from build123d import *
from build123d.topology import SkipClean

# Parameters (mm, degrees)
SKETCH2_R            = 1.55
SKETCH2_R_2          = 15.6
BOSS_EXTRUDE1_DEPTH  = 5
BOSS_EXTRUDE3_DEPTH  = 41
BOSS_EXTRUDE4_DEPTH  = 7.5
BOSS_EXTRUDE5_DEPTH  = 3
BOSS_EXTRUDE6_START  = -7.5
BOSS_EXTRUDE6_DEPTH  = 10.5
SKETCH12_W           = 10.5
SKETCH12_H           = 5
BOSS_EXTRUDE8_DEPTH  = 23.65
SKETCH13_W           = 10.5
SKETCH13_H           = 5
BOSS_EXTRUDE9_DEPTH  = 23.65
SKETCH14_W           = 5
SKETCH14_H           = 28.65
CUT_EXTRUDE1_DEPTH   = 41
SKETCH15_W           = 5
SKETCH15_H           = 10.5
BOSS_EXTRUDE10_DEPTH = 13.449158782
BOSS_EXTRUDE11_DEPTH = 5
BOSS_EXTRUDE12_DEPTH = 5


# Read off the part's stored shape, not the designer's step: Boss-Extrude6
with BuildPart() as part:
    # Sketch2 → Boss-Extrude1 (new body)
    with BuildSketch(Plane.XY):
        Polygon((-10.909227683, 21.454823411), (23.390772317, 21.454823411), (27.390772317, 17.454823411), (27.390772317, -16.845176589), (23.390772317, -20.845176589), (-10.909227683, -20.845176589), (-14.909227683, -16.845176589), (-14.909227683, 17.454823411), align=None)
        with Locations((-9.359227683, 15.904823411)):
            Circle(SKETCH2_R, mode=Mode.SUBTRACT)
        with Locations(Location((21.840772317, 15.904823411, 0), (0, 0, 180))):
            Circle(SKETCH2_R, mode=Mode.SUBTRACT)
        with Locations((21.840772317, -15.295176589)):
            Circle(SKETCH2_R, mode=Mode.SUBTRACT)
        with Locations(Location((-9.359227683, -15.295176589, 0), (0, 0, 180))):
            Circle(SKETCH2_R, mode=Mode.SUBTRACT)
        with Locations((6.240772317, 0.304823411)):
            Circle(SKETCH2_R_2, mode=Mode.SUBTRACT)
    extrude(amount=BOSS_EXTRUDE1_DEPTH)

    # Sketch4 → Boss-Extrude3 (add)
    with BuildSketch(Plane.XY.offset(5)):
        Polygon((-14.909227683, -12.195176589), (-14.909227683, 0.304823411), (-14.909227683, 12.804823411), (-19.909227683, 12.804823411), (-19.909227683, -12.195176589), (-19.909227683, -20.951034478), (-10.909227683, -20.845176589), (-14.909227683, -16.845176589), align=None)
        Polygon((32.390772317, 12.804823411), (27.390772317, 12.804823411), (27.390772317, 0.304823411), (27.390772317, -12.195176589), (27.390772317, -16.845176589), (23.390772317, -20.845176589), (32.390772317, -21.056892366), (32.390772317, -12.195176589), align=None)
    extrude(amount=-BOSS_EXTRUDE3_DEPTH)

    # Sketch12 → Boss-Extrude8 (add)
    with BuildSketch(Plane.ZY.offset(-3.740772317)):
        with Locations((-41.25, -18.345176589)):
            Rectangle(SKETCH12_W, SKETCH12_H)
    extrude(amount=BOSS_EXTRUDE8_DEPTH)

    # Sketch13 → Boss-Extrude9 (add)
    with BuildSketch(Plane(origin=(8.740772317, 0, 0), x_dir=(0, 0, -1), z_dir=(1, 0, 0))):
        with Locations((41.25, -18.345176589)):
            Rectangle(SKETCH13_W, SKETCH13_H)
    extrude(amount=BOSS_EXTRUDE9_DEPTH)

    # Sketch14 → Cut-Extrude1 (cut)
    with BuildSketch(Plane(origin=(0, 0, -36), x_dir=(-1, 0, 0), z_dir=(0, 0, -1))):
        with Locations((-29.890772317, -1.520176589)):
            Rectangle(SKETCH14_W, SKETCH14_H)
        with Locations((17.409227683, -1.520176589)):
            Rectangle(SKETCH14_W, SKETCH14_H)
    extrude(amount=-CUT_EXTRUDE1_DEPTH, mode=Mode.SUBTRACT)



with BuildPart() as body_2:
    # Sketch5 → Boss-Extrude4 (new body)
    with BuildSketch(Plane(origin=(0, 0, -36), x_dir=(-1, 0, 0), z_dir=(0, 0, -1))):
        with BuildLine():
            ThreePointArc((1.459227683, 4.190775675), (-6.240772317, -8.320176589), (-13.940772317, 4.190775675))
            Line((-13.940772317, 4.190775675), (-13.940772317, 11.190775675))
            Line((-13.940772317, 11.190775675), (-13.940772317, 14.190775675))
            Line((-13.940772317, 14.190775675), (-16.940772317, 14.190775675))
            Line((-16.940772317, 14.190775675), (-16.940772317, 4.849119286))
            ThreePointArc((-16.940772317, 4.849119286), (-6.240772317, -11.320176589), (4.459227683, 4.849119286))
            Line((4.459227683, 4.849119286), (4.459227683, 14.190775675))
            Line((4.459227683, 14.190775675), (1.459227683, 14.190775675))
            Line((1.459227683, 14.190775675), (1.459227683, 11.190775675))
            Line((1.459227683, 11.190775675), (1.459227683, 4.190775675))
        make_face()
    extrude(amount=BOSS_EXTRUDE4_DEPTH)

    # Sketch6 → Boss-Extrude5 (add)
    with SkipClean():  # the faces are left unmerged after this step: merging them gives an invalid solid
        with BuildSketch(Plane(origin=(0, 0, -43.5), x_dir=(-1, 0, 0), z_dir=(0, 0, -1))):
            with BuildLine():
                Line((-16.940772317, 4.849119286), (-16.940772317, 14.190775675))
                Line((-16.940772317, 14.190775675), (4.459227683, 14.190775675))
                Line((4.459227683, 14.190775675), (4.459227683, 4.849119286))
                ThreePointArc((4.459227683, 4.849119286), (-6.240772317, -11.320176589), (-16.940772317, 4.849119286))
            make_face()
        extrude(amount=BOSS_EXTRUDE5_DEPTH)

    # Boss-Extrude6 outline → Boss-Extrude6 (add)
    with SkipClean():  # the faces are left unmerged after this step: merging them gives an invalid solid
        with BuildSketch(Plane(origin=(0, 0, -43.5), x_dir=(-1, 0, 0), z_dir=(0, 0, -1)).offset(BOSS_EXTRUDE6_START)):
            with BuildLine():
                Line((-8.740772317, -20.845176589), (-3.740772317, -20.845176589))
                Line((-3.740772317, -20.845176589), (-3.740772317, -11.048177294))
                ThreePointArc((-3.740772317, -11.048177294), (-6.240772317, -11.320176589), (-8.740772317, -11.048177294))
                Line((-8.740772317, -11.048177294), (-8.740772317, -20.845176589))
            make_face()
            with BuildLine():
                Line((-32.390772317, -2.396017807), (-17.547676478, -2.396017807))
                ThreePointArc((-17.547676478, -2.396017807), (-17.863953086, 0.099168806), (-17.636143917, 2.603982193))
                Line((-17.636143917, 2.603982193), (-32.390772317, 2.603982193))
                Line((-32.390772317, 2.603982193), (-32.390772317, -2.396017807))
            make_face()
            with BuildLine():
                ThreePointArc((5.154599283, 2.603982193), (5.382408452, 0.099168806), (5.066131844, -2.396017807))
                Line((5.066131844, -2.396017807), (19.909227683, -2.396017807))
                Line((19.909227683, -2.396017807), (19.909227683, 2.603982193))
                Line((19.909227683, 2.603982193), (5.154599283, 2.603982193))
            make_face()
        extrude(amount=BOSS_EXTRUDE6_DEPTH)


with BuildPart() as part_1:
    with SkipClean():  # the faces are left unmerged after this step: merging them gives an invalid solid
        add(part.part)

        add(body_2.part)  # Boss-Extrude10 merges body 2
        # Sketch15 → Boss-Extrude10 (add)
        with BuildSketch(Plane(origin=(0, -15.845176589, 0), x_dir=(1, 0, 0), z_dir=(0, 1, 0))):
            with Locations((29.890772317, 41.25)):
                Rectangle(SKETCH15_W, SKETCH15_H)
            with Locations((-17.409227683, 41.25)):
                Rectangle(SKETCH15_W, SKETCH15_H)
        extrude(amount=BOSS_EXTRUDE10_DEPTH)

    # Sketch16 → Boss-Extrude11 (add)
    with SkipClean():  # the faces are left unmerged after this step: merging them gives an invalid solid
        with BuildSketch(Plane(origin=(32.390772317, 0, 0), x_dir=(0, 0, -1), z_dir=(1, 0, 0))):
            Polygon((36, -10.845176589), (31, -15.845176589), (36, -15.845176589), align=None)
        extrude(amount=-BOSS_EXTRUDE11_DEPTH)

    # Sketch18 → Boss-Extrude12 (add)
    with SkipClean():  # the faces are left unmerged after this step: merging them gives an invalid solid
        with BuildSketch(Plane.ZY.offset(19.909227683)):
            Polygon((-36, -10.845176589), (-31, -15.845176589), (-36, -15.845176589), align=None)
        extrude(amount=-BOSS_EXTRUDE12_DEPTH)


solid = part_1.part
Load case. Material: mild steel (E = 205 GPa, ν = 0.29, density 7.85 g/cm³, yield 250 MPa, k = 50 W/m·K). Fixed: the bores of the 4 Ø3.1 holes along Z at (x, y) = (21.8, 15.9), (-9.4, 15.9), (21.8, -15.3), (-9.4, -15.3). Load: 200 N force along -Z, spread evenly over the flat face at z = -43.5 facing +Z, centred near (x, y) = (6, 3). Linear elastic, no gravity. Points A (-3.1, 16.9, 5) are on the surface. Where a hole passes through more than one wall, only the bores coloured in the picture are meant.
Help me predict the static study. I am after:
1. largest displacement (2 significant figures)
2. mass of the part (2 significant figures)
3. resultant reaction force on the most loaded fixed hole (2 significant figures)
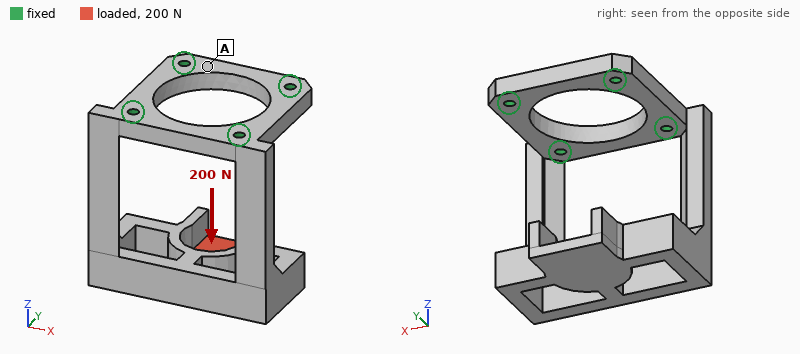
0.31 mm
130 g
94 N
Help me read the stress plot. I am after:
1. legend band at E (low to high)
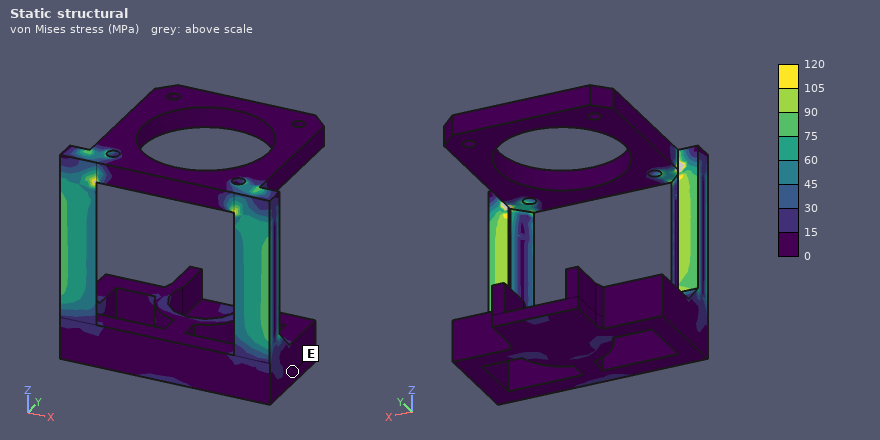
0 to 15 MPa
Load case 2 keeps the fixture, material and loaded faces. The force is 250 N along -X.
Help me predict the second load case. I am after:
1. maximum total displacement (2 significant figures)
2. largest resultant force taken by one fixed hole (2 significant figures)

0.16 mm
240 N
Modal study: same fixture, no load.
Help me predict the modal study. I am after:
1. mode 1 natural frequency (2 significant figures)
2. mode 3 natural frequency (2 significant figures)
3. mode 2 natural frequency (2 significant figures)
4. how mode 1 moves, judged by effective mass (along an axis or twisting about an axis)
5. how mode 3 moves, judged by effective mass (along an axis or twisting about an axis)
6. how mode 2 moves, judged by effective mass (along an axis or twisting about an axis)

460 Hz
1900 Hz
930 Hz
along Y
along X
along X
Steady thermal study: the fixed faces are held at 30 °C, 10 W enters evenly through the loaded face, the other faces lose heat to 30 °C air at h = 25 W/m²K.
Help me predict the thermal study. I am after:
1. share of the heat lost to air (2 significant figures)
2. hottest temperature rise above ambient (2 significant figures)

74 %
69 K
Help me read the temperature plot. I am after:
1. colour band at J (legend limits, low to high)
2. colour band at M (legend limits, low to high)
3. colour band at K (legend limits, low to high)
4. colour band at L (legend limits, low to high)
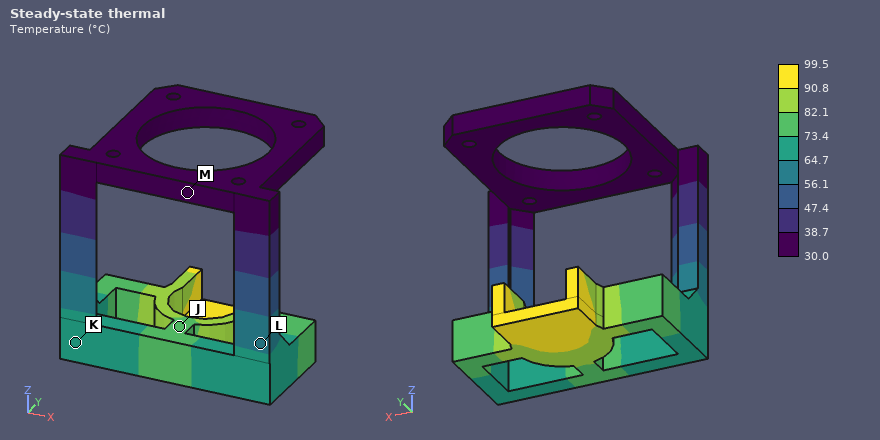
73.4 to 82.1 °C
30.0 to 38.7 °C
64.7 to 73.4 °C
56.1 to 64.7 °C
